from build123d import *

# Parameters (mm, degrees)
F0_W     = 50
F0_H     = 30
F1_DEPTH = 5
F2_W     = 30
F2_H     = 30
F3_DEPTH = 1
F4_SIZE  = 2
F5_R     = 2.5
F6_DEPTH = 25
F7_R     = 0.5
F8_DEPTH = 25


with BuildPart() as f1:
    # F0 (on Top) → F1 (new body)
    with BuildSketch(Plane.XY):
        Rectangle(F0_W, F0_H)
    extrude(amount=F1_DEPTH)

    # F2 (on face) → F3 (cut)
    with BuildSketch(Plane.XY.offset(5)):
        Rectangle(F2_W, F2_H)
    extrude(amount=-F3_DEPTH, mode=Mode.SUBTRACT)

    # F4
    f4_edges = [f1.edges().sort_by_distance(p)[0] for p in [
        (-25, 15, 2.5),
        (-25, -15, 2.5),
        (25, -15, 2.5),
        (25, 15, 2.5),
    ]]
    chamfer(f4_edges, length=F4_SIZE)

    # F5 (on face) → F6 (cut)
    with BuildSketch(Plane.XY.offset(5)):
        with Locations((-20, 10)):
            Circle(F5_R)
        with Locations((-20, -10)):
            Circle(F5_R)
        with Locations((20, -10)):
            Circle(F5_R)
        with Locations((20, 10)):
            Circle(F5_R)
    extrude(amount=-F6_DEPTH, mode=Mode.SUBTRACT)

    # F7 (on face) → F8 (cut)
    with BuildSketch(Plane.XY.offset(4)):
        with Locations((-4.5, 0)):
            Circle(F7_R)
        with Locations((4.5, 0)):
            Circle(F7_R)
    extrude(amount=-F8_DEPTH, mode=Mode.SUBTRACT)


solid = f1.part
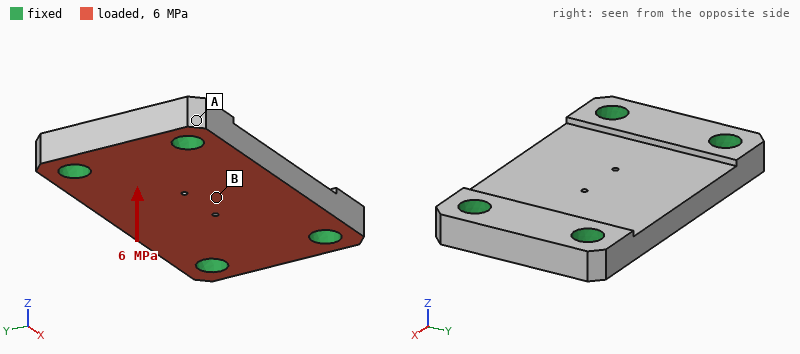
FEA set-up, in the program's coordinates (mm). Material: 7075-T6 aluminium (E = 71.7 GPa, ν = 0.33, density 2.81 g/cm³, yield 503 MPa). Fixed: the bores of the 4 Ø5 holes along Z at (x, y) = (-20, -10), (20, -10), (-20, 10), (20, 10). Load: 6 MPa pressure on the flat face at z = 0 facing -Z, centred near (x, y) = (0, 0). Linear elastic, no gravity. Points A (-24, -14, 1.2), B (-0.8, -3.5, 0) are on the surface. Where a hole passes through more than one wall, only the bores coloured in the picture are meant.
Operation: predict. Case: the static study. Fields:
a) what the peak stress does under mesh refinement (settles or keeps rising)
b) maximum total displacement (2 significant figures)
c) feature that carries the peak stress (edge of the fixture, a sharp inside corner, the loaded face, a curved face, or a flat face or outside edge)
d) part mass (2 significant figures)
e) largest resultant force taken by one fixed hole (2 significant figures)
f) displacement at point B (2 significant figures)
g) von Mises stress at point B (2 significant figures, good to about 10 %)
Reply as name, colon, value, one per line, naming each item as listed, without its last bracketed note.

what the peak stress does under mesh refinement: keeps rising
maximum total displacement: 78 µm
feature that carries the peak stress: edge of the fixture
part mass: 17 g
largest resultant force taken by one fixed hole: 2.2 kN
displacement at point B: 75 µm
von Mises stress at point B: 110 MPa
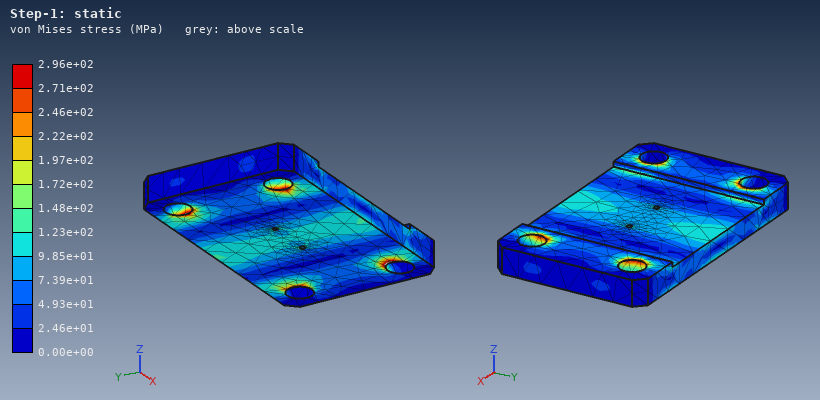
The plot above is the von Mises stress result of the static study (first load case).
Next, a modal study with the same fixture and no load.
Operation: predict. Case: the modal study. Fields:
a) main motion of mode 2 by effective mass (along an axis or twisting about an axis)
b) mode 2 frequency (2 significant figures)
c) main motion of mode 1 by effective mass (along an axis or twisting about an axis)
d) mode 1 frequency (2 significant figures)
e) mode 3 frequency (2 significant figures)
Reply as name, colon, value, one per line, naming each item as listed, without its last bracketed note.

main motion of mode 2 by effective mass: twisting about X
mode 2 frequency: 19 kHz
main motion of mode 1 by effective mass: along Z
mode 1 frequency: 15 kHz
mode 3 frequency: 33 kHz
